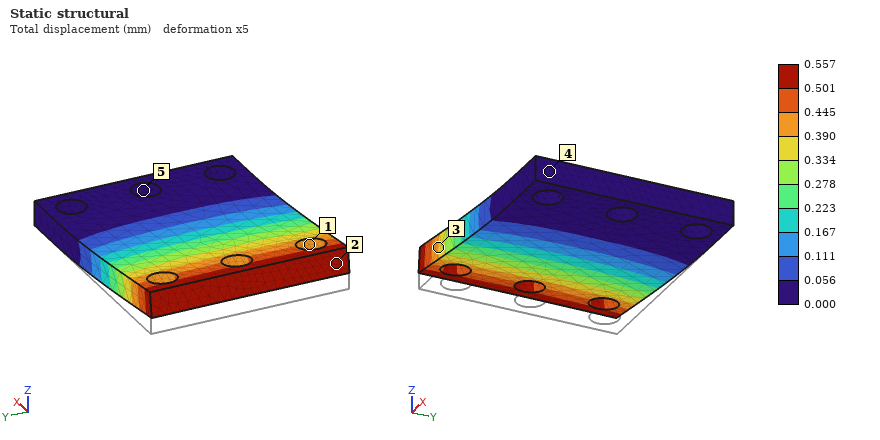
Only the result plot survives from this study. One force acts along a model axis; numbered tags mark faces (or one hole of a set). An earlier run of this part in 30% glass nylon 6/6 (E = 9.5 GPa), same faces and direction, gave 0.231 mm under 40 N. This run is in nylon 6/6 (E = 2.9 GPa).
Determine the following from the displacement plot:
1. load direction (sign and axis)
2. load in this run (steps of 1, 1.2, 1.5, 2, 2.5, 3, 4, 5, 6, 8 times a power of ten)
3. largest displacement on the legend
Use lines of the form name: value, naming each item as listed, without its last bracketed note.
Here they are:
load direction: +Z
load in this run: 30 N
largest displacement on the legend: 0.557 mm
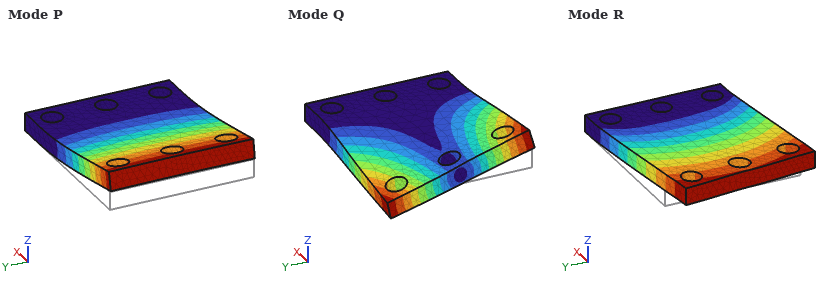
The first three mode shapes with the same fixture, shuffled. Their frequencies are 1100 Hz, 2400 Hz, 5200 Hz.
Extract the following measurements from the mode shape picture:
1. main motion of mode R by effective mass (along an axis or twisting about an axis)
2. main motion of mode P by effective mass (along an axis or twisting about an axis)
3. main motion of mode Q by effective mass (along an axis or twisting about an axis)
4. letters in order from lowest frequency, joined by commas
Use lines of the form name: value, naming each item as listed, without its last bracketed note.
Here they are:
main motion of mode R by effective mass: along Y
main motion of mode P by effective mass: along Z
main motion of mode Q by effective mass: twisting about X
letters in order from lowest frequency, joined by commas: P, Q, R
